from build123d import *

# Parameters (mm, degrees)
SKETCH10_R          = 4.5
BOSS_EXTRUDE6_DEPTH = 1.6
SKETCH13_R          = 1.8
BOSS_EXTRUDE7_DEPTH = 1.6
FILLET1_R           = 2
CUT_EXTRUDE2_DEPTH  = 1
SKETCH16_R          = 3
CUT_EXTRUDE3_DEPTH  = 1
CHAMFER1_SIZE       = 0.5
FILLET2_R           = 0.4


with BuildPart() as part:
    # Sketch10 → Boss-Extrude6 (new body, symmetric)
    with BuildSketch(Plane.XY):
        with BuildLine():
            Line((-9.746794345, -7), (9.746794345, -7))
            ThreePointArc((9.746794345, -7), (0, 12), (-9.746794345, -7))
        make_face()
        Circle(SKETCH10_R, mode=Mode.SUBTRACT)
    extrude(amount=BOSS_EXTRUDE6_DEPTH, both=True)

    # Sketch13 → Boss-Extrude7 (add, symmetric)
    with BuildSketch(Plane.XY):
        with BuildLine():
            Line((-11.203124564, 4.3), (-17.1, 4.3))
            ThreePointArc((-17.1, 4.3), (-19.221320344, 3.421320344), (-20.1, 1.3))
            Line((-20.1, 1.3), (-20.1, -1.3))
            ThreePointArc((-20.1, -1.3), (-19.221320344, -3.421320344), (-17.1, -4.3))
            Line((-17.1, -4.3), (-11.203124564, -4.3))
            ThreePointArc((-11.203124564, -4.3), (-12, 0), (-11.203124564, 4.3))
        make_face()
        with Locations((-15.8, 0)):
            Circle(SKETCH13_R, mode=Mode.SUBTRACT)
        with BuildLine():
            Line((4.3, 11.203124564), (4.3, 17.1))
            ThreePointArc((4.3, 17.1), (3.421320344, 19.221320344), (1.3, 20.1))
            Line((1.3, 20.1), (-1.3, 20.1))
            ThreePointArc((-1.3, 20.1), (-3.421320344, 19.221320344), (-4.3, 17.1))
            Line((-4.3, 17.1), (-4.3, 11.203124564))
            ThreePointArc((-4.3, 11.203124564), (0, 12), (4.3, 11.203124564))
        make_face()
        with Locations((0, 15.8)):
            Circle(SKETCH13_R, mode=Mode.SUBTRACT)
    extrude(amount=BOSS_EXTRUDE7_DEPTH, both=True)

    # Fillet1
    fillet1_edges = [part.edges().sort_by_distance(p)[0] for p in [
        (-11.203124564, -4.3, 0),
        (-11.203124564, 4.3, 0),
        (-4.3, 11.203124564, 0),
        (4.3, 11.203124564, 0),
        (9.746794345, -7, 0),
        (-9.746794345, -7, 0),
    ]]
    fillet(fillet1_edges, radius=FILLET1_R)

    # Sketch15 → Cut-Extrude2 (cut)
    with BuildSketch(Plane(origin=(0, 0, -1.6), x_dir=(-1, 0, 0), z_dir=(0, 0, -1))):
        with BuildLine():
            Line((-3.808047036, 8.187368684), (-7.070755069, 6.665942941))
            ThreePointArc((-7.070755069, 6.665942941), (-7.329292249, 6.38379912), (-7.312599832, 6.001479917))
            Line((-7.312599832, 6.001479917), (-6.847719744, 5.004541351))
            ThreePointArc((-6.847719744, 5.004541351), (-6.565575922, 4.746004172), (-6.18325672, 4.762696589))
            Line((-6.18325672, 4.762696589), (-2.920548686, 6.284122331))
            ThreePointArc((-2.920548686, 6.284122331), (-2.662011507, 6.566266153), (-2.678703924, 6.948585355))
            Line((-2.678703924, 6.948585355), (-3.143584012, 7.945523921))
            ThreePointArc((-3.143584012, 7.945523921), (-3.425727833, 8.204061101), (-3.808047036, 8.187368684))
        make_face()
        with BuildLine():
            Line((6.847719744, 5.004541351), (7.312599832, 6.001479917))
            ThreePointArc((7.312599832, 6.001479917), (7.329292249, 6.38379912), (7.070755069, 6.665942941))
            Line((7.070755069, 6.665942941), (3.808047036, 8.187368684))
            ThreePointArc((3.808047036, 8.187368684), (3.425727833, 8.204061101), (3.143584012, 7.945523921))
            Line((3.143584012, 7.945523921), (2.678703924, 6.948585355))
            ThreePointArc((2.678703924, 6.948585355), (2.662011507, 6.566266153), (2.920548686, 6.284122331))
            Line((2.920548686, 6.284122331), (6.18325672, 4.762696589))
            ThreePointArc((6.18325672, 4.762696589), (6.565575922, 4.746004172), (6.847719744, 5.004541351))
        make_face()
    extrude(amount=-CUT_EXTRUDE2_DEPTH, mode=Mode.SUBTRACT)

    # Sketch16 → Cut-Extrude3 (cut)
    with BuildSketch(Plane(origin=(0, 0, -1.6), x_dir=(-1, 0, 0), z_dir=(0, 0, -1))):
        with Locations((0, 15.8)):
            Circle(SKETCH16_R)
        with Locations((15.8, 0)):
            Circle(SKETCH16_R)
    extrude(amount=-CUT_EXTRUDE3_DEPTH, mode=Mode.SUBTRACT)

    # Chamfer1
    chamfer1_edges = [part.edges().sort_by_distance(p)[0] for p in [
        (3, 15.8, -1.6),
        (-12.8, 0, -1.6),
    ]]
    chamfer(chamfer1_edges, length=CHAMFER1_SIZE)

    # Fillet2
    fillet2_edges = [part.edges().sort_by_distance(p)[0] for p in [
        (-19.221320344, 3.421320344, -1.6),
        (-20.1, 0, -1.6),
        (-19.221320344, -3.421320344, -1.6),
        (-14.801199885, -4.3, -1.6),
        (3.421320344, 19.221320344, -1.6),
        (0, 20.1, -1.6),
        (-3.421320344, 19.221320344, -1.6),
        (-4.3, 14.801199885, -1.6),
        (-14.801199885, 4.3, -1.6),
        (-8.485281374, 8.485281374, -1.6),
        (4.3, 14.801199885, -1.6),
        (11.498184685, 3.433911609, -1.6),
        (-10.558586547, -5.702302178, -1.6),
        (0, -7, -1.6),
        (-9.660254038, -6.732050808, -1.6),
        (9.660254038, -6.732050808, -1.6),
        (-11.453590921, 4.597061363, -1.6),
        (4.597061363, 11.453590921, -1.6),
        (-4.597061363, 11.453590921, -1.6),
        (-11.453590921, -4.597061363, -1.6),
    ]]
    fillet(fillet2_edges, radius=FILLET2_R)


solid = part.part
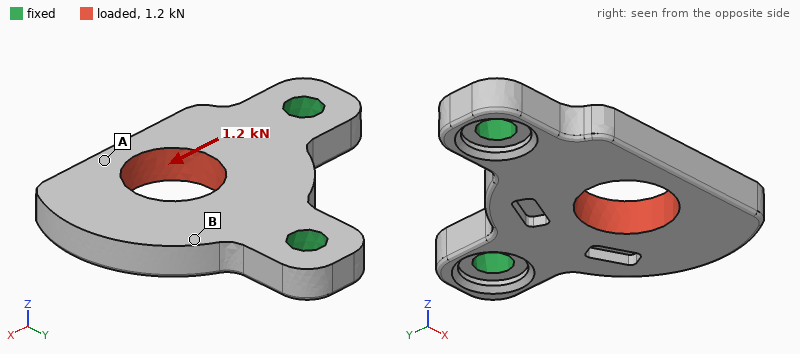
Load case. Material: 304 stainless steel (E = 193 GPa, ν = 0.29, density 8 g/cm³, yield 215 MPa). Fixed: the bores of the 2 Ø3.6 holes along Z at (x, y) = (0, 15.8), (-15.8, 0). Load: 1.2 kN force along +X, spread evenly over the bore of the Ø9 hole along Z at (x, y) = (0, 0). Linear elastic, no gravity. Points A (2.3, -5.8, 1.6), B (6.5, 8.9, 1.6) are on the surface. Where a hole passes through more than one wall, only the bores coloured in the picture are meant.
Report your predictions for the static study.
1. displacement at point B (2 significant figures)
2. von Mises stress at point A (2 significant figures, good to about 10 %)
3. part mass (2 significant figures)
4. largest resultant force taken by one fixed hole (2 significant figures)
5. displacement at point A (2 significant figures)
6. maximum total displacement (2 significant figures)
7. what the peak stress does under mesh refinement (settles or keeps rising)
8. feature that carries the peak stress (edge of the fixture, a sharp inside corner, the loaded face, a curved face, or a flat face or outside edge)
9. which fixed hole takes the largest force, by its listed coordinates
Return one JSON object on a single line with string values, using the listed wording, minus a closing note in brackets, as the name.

{"displacement at point B": "3.0 µm", "von Mises stress at point A": "27 MPa", "part mass": "11 g", "largest resultant force taken by one fixed hole": "1.0 kN", "displacement at point A": "6.1 µm", "maximum total displacement": "7.2 µm", "what the peak stress does under mesh refinement": "keeps rising", "feature that carries the peak stress": "edge of the fixture", "which fixed hole takes the largest force, by its listed coordinates": "(-15.8, 0)"}
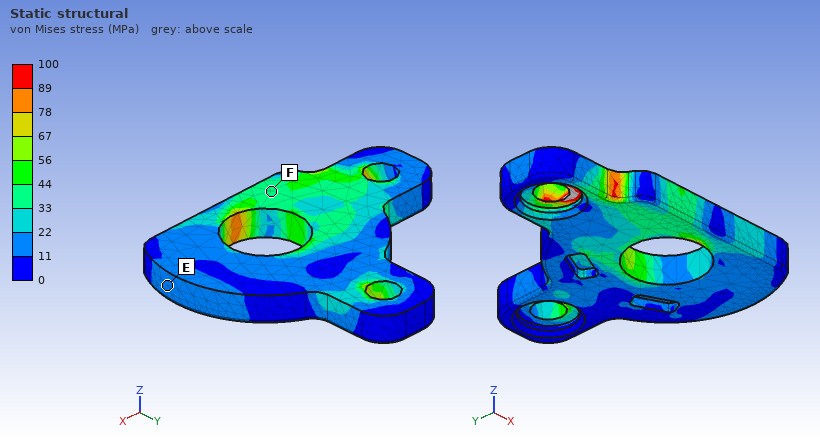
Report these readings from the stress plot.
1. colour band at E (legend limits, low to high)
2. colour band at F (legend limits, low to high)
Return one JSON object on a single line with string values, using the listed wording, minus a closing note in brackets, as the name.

{"colour band at E": "11 to 22 MPa", "colour band at F": "33 to 44 MPa"}
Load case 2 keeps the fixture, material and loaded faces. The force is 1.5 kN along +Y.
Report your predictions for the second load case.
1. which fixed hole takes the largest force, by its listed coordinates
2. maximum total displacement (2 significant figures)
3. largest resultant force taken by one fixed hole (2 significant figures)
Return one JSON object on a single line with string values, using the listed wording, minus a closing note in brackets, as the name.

{"which fixed hole takes the largest force, by its listed coordinates": "(0, 15.8)", "maximum total displacement": "9.5 µm", "largest resultant force taken by one fixed hole": "1.3 kN"}
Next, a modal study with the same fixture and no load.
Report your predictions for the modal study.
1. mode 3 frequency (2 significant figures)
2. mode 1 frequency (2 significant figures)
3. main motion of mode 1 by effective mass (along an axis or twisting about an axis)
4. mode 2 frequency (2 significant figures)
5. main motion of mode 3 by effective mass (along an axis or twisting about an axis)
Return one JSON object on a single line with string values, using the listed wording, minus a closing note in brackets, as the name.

{"mode 3 frequency": "24 kHz", "mode 1 frequency": "5300 Hz", "main motion of mode 1 by effective mass": "along Z", "mode 2 frequency": "17 kHz", "main motion of mode 3 by effective mass": "along Z"}
